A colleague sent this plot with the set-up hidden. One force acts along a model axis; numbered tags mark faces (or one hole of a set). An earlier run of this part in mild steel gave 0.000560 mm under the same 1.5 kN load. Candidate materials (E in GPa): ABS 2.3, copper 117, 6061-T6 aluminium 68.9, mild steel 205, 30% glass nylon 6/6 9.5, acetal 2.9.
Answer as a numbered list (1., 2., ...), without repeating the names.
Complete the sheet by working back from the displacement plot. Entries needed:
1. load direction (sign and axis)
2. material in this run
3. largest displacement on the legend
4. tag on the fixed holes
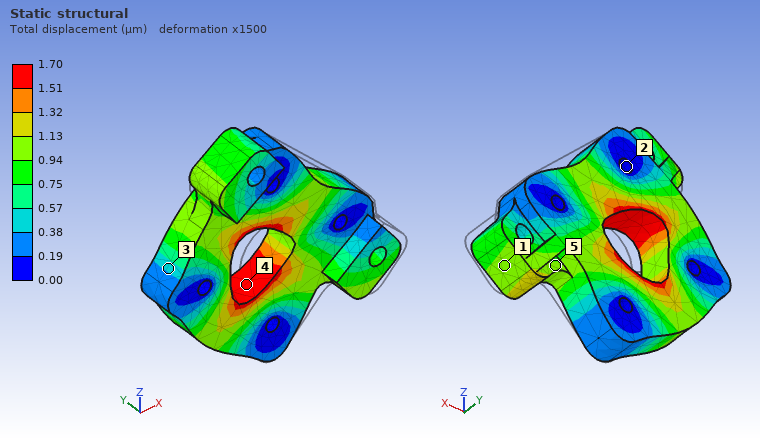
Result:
1. -X
2. 6061-T6 aluminium
3. 1.70 µm
4. 2
